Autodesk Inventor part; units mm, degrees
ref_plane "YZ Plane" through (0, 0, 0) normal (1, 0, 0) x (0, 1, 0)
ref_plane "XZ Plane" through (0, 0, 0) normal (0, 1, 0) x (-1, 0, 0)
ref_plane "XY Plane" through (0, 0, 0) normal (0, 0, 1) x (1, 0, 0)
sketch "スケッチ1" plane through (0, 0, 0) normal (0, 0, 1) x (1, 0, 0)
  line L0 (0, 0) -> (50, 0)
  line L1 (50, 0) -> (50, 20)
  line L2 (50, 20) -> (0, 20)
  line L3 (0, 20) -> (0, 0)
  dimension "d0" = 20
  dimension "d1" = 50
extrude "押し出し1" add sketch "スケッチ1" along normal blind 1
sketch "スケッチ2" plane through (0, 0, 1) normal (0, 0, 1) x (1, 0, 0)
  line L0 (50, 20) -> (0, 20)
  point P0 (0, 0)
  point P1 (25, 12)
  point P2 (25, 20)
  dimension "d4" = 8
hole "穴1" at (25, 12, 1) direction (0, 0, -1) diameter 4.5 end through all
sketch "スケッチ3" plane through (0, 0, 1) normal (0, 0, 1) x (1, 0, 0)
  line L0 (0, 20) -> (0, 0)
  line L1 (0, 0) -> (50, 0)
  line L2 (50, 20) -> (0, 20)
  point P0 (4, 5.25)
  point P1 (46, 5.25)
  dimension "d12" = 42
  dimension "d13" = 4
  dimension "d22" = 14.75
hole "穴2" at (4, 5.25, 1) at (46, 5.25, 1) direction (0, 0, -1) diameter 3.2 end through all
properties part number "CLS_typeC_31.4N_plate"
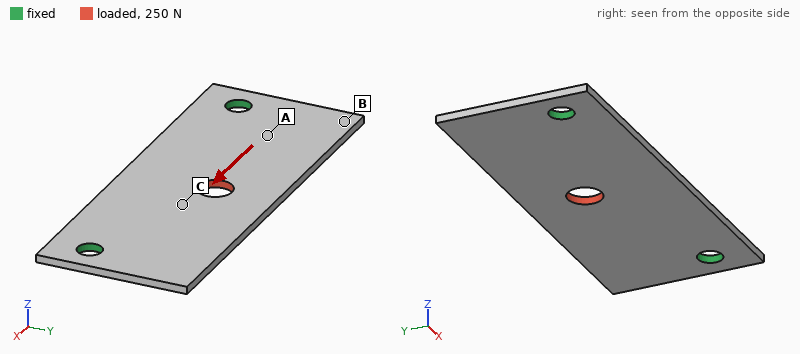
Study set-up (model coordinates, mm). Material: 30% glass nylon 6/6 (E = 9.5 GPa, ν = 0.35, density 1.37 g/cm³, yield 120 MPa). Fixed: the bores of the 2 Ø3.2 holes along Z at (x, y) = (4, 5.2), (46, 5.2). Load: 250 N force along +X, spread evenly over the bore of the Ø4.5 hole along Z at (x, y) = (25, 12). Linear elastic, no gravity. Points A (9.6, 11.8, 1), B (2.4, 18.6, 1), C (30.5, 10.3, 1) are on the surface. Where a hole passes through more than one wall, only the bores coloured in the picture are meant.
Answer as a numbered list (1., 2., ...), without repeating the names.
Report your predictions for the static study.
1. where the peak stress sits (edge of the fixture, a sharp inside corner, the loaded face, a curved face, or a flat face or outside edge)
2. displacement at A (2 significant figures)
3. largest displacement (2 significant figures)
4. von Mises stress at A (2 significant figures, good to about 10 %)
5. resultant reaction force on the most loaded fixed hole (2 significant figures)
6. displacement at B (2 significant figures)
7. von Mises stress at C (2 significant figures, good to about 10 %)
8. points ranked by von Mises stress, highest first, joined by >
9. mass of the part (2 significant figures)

1. edge of the fixture
2. 14 µm
3. 32 µm
4. 8.1 MPa
5. 130 N
6. 20 µm
7. 14 MPa
8. C > A > B
9. 1.3 g
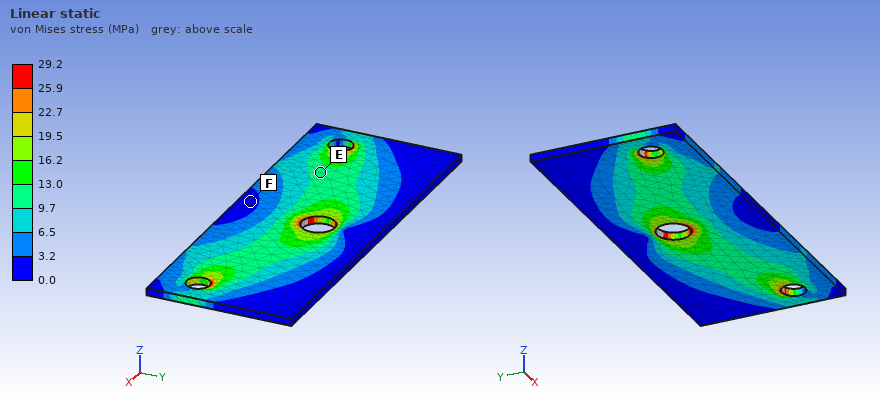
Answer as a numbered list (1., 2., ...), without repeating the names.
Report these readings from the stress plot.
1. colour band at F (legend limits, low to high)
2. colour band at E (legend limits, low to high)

1. 0.0 to 3.2 MPa
2. 9.7 to 13.0 MPa
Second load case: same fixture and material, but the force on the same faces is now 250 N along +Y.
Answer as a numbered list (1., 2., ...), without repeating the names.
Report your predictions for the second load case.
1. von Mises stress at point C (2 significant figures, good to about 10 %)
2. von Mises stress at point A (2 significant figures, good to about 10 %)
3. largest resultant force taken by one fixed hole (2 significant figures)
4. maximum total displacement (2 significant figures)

1. 13 MPa
2. 15 MPa
3. 150 N
4. 84 µm
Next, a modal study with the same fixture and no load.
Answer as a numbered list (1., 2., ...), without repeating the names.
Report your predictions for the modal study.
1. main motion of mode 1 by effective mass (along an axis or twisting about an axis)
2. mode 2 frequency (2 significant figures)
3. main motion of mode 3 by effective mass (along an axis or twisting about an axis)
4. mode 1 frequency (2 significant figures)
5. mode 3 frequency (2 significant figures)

1. along Z
2. 2000 Hz
3. twisting about Y
4. 1200 Hz
5. 2400 Hz
